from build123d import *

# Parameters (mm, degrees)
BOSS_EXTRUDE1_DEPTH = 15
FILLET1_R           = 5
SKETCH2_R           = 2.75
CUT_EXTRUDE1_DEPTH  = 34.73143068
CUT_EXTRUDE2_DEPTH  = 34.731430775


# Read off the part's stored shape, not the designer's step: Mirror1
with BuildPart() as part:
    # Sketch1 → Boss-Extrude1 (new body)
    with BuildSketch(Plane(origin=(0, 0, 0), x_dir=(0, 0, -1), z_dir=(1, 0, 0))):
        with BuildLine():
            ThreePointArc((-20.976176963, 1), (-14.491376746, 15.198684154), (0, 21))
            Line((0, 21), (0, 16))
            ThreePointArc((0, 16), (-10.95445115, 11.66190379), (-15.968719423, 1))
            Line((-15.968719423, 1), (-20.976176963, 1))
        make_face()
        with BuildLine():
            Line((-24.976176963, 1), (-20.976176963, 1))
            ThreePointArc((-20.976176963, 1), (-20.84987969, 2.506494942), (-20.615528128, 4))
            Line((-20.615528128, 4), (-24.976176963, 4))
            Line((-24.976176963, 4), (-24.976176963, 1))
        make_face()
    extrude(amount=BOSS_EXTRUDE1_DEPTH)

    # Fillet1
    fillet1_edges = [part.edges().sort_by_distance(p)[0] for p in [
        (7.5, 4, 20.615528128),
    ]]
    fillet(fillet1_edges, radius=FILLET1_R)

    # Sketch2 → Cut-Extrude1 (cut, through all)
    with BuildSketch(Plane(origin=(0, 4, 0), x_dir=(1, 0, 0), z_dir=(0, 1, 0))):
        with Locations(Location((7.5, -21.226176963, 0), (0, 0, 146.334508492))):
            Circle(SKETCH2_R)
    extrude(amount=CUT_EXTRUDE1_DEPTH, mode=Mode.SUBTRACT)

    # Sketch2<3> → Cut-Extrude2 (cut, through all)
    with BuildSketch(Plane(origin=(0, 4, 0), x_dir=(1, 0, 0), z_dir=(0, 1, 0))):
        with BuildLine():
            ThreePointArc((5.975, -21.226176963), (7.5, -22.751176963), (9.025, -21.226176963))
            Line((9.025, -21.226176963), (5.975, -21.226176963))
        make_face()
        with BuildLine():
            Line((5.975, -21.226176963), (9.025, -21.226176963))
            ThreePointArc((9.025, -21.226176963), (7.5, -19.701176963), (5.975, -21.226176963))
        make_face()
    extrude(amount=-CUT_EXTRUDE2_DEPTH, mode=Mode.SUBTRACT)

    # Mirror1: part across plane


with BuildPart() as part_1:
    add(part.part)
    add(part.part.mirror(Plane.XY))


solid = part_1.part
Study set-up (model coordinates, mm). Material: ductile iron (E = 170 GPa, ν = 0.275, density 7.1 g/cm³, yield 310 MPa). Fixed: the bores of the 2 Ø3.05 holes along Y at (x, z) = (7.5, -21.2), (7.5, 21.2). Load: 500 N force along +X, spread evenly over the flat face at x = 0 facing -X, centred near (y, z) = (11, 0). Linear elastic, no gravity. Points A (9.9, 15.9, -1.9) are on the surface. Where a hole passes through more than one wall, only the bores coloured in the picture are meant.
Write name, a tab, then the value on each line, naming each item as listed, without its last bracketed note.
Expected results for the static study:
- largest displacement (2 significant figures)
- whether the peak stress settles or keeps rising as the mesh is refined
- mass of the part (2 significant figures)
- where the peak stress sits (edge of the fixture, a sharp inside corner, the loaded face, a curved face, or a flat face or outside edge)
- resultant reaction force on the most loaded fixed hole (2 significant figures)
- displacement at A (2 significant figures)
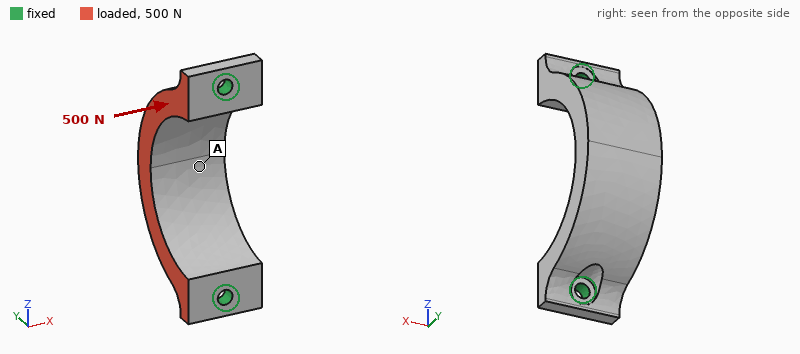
largest displacement	17 µm
whether the peak stress settles or keeps rising as the mesh is refined	keeps rising
mass of the part	32 g
where the peak stress sits	edge of the fixture
resultant reaction force on the most loaded fixed hole	250 N
displacement at A	12 µm
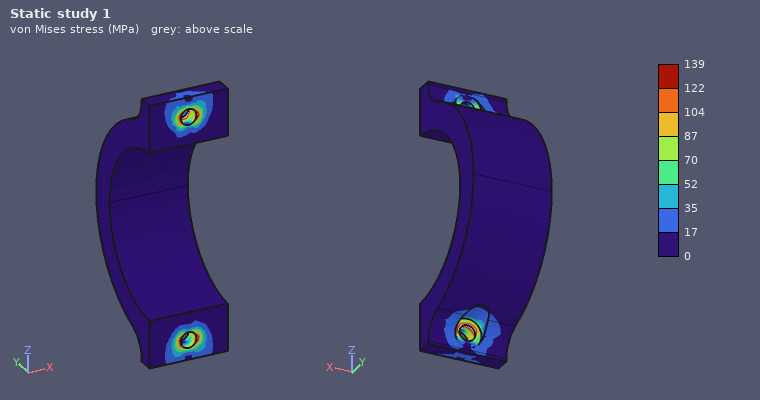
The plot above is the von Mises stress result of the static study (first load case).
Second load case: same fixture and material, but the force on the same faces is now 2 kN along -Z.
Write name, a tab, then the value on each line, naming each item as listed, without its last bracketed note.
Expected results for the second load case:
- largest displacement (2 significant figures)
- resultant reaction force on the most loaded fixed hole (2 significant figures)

largest displacement	19 µm
resultant reaction force on the most loaded fixed hole	1.1 kN
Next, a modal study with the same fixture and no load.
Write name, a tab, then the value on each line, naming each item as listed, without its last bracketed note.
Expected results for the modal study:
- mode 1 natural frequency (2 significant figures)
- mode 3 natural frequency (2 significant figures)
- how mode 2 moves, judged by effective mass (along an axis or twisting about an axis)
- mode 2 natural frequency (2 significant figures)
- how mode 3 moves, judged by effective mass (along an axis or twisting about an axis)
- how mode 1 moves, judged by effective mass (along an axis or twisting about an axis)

mode 1 natural frequency	5700 Hz
mode 3 natural frequency	17 kHz
how mode 2 moves, judged by effective mass	along Z
mode 2 natural frequency	12 kHz
how mode 3 moves, judged by effective mass	twisting about Y
how mode 1 moves, judged by effective mass	along X
